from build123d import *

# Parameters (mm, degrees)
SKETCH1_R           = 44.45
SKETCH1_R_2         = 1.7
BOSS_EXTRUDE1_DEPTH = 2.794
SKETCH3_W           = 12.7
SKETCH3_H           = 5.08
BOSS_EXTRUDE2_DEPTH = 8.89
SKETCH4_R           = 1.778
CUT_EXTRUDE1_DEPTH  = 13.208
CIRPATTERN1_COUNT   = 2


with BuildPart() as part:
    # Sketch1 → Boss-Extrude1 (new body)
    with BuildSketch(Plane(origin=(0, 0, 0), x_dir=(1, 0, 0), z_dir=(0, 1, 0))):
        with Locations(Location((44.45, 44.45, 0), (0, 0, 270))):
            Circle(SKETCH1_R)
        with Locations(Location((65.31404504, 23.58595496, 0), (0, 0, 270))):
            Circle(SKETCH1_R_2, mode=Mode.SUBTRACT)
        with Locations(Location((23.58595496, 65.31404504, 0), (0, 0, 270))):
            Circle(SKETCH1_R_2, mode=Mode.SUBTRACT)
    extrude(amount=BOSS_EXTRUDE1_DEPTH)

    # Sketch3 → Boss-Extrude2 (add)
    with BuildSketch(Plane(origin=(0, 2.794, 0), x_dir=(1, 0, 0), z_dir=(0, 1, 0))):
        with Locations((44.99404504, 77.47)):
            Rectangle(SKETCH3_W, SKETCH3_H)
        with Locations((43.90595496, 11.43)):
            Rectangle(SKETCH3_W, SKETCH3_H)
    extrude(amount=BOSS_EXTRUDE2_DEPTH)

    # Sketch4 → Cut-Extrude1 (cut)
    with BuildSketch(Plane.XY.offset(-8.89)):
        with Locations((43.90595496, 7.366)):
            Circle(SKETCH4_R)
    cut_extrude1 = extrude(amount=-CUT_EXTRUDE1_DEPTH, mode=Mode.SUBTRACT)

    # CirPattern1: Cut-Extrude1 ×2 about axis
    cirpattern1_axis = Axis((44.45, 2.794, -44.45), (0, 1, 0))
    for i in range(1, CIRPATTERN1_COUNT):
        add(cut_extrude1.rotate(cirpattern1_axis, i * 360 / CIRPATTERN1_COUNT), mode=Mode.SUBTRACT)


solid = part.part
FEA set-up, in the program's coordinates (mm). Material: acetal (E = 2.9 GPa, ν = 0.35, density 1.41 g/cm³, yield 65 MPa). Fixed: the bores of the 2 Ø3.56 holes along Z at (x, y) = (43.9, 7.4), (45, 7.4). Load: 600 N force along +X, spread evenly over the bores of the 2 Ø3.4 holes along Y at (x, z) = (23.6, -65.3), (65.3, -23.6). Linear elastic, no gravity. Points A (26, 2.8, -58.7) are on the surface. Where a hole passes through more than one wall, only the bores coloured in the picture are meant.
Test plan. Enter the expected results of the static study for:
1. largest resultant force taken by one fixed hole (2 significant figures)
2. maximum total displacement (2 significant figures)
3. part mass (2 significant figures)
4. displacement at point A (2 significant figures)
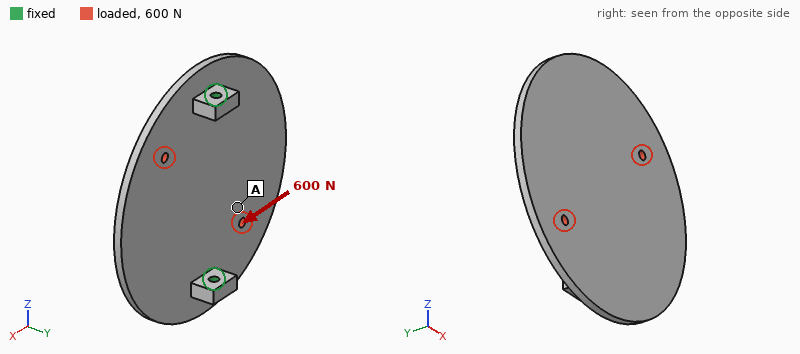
300 N
0.45 mm
26 g
0.21 mm
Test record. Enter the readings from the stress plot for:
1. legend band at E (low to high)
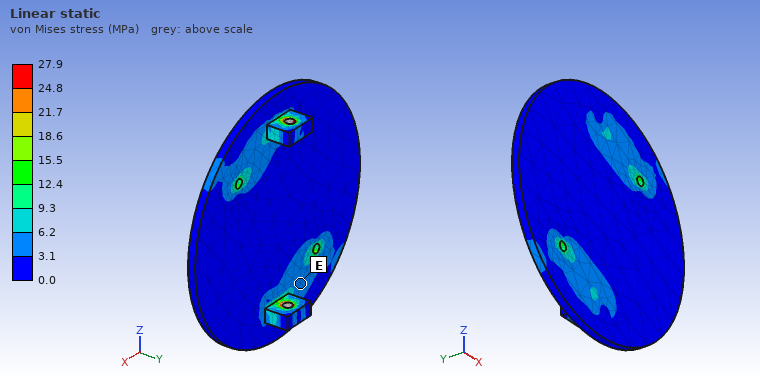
3.1 to 6.2 MPa
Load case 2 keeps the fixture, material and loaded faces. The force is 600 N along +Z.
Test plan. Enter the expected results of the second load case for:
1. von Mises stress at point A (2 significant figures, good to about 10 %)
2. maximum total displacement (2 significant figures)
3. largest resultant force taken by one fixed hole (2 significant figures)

4.6 MPa
0.14 mm
300 N
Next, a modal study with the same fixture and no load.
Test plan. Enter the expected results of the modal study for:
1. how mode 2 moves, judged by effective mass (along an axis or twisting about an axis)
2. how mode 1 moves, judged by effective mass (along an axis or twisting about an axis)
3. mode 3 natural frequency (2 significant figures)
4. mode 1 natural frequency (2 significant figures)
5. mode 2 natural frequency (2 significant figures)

along Y
twisting about Z
910 Hz
340 Hz
420 Hz
